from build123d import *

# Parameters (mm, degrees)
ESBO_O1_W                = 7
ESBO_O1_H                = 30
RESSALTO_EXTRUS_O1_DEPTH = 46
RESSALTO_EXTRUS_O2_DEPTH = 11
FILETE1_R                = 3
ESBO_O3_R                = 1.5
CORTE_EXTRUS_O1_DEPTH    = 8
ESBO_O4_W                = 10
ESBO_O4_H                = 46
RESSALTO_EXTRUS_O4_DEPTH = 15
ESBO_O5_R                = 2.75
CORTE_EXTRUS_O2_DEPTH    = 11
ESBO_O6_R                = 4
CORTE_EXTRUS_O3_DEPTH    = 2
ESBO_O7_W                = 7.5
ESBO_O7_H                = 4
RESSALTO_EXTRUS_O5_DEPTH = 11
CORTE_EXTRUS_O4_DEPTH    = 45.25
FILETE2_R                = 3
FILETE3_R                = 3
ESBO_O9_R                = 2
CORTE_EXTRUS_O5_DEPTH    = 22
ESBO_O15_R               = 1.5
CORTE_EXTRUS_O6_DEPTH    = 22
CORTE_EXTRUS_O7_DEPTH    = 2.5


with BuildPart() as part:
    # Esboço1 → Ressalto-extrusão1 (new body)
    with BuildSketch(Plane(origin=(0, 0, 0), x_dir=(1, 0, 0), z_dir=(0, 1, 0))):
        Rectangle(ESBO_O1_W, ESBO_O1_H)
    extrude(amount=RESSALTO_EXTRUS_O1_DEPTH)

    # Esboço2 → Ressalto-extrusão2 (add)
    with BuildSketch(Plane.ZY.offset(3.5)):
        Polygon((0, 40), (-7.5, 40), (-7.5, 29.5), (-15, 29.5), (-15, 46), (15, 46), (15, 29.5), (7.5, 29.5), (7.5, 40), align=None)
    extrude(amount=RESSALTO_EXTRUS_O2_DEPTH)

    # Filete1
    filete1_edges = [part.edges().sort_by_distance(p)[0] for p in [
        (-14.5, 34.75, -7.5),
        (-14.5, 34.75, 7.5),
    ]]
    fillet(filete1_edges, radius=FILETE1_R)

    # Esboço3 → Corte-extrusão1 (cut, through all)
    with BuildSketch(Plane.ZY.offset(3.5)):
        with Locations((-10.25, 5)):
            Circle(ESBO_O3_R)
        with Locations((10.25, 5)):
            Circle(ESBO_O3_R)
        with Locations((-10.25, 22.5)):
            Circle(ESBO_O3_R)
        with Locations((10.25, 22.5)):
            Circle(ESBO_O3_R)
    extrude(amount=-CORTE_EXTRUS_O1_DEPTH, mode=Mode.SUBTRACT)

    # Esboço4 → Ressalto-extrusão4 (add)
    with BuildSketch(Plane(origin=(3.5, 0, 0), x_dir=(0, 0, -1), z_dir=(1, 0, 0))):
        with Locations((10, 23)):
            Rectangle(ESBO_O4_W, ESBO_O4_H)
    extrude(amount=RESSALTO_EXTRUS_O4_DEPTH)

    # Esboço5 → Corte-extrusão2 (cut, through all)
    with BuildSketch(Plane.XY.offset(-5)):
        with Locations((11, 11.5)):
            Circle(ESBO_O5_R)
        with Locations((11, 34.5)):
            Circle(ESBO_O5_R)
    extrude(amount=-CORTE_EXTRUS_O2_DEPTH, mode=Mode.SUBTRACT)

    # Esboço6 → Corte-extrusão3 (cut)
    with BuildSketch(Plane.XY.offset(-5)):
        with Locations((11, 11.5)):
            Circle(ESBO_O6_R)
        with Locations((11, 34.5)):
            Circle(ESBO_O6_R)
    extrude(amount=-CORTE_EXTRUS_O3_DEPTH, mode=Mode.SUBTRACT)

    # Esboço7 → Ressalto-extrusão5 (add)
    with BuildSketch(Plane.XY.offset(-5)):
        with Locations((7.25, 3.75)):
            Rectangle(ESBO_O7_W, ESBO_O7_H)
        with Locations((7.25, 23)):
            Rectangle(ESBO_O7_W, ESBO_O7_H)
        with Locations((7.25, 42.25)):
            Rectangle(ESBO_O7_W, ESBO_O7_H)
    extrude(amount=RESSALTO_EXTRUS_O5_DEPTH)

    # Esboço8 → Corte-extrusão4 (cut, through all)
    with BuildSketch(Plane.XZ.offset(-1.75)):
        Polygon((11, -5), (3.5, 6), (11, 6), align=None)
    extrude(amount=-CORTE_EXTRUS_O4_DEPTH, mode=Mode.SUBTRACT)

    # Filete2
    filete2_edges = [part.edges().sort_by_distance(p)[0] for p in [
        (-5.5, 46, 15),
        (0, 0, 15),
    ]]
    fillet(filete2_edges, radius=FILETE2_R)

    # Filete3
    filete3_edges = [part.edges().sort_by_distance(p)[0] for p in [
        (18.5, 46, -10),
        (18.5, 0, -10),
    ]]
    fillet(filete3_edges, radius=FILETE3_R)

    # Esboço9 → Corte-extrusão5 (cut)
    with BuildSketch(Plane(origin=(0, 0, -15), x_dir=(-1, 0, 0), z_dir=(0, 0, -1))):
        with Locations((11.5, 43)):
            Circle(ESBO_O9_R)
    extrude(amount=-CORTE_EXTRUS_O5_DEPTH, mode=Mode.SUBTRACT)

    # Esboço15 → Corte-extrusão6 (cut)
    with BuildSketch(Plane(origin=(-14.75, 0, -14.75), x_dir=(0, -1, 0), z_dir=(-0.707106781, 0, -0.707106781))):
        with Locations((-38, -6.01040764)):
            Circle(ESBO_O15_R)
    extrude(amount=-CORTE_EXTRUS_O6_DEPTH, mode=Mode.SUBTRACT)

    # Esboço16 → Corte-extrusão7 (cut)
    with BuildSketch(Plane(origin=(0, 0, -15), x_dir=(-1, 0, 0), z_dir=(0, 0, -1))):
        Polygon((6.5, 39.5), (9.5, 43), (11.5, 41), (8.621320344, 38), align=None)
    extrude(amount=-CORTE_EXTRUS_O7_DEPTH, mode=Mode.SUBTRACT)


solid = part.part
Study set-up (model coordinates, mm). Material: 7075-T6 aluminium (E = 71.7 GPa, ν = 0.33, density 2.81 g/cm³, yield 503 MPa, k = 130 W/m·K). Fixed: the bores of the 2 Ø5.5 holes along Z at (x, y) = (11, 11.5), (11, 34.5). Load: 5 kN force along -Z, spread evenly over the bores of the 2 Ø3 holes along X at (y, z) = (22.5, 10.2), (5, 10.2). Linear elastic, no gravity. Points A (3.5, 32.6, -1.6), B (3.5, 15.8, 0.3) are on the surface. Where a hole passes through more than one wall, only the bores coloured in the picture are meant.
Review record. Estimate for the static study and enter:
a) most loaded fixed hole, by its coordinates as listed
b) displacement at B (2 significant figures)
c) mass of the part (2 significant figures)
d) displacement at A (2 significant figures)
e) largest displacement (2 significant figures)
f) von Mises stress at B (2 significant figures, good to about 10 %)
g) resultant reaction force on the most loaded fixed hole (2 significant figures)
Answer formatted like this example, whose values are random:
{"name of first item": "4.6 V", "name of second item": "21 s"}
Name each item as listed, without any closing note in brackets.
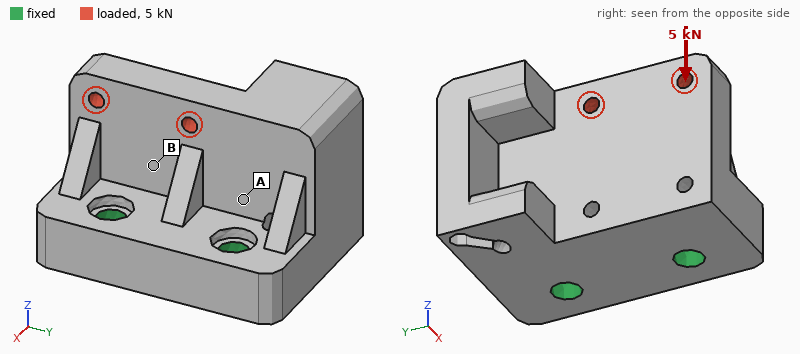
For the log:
{"most loaded fixed hole, by its coordinates as listed": "(11, 11.5)", "displacement at B": "29 µm", "mass of the part": "55 g", "displacement at A": "16 µm", "largest displacement": "79 µm", "von Mises stress at B": "29 MPa", "resultant reaction force on the most loaded fixed hole": "4.0 kN"}
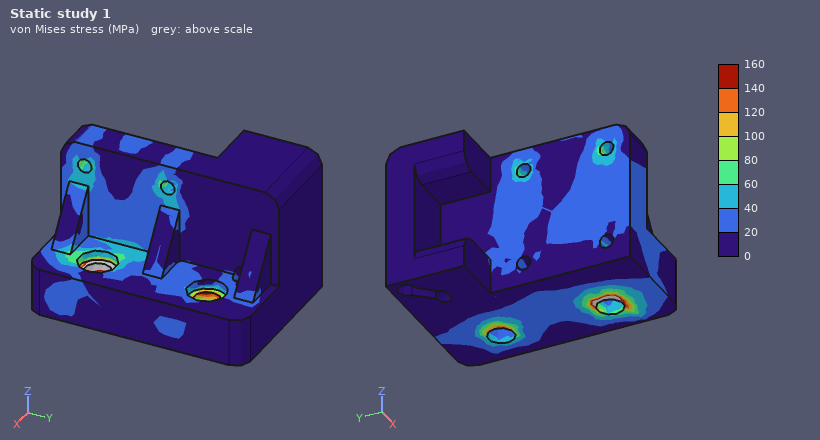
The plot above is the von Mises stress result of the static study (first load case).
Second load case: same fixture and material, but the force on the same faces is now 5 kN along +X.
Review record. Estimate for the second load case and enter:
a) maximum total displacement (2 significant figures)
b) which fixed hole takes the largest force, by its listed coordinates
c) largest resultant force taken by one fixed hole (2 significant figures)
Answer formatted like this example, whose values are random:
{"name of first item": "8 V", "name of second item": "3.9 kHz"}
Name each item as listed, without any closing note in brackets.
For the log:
{"maximum total displacement": "0.25 mm", "which fixed hole takes the largest force, by its listed coordinates": "(11, 11.5)", "largest resultant force taken by one fixed hole": "4.2 kN"}
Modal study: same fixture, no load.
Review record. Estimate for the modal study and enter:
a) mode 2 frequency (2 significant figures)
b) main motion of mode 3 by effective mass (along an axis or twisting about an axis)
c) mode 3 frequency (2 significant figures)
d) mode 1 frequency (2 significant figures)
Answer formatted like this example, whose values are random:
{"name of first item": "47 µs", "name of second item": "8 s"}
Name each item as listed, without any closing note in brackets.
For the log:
{"mode 2 frequency": "11 kHz", "main motion of mode 3 by effective mass": "along Y", "mode 3 frequency": "13 kHz", "mode 1 frequency": "6200 Hz"}
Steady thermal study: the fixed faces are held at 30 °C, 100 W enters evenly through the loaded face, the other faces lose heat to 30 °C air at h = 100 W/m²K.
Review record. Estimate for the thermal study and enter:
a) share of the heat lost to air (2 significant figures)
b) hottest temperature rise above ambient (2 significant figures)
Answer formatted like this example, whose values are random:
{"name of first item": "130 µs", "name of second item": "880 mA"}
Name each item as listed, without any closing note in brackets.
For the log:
{"share of the heat lost to air": "15 %", "hottest temperature rise above ambient": "80 K"}
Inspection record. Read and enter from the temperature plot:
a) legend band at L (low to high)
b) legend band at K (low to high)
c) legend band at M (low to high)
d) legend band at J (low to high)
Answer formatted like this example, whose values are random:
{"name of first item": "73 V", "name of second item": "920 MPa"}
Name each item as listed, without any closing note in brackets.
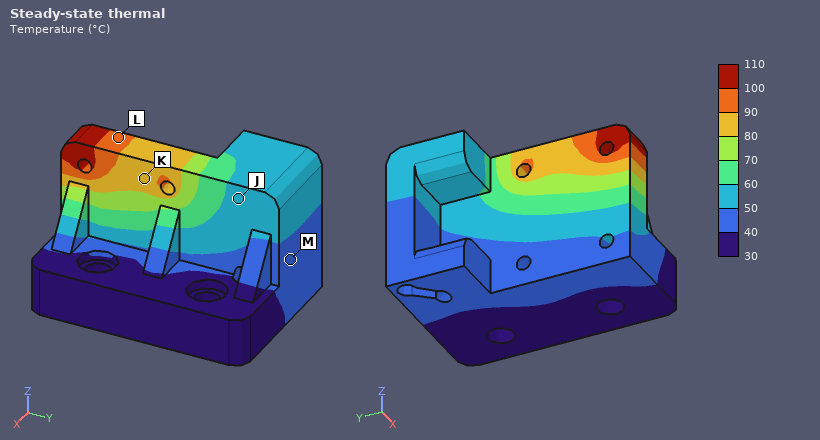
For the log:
{"legend band at L": "90 to 100 °C", "legend band at K": "80 to 90 °C", "legend band at M": "40 to 50 °C", "legend band at J": "50 to 60 °C"}
